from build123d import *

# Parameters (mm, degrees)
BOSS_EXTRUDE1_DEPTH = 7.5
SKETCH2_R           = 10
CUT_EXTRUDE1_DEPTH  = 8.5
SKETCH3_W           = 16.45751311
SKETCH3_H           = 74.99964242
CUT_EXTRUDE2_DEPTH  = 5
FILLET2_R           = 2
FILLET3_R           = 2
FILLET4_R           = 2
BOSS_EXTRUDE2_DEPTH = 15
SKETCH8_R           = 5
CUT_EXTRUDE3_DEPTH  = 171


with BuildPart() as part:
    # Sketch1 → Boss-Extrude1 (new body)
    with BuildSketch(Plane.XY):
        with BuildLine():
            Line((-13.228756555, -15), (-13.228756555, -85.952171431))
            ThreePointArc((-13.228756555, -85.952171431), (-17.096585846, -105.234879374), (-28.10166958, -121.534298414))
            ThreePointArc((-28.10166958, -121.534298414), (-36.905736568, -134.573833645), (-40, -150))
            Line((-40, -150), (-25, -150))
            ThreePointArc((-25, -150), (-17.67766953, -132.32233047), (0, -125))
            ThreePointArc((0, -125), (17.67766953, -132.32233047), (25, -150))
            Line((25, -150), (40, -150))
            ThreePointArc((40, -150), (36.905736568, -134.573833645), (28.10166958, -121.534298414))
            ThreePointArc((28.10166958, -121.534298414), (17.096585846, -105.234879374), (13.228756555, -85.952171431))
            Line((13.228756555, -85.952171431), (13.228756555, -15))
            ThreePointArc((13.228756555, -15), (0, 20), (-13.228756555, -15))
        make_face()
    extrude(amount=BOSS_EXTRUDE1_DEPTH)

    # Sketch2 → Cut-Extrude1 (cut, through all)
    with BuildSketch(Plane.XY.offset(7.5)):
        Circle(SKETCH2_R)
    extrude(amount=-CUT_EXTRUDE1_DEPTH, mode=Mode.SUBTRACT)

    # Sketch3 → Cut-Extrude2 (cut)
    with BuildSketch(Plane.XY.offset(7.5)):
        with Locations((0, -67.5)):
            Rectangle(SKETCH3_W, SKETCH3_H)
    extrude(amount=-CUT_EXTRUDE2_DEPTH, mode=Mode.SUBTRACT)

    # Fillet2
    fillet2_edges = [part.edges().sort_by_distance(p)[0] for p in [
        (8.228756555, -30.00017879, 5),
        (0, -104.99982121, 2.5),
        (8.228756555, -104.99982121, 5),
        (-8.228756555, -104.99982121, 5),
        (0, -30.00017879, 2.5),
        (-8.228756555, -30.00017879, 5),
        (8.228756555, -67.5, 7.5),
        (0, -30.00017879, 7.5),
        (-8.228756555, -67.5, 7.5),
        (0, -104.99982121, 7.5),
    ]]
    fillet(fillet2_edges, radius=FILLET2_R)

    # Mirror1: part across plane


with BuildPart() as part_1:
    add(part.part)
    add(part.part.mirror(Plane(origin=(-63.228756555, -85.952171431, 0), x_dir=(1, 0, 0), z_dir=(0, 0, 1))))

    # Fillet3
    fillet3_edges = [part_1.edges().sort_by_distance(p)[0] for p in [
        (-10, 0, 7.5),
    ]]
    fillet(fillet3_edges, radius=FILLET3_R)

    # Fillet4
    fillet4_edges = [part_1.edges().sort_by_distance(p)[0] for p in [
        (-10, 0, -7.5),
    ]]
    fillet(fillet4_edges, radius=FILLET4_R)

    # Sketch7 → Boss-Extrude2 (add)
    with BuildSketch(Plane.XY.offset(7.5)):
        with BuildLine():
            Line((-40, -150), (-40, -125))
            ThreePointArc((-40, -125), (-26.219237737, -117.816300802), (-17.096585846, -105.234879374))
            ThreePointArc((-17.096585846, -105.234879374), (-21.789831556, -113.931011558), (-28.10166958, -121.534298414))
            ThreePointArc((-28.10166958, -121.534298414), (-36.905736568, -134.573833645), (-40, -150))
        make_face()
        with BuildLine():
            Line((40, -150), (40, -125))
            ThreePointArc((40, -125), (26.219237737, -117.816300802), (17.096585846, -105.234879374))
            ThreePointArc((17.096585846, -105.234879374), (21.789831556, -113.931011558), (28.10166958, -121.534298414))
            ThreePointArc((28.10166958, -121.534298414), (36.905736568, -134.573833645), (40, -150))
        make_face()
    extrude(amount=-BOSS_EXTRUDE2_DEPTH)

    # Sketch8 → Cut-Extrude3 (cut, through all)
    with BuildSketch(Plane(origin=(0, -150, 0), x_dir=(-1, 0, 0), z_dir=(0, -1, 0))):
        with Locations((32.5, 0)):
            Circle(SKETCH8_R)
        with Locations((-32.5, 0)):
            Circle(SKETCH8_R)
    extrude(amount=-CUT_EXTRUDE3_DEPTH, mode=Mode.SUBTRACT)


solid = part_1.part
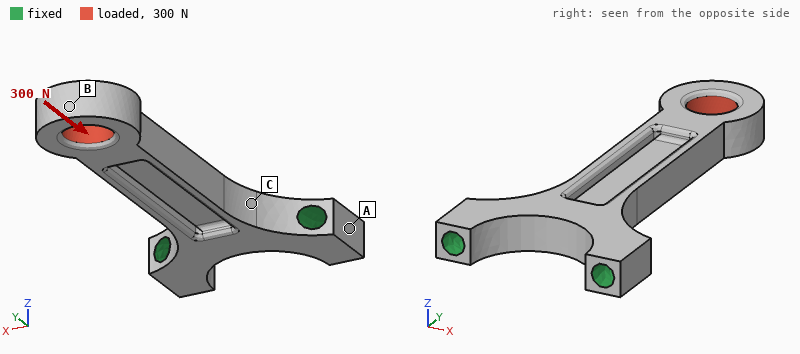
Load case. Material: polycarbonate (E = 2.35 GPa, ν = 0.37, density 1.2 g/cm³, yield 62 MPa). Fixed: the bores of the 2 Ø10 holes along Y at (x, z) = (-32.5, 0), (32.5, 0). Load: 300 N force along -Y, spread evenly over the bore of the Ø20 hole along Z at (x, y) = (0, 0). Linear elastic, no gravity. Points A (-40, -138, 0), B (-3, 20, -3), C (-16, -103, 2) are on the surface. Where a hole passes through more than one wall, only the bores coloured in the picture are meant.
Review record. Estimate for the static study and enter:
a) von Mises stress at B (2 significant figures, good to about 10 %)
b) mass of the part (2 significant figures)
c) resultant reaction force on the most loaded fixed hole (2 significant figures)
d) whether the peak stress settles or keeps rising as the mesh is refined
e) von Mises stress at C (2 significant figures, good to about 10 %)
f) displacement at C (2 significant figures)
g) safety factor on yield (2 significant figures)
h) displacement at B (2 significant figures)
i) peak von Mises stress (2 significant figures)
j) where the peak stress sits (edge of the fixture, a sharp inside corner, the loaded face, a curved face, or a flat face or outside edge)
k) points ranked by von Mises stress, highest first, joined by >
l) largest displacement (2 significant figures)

0.79 MPa
75 g
180 N
settles
1.2 MPa
13 µm
26
76 µm
2.4 MPa
the loaded face
C > B > A
78 µm
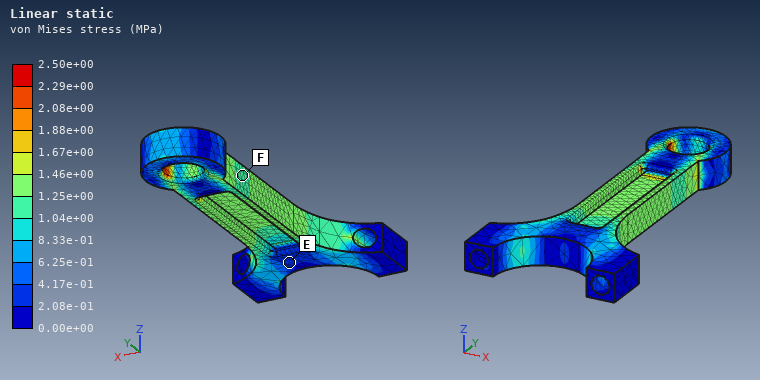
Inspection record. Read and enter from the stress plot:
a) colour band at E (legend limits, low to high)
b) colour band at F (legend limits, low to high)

2.08e-01 to 4.17e-01 MPa
1.04e+00 to 1.25e+00 MPa
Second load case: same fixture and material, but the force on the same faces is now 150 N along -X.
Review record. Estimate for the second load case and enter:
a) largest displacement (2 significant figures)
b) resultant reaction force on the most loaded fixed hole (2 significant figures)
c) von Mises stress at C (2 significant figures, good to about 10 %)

2.0 mm
410 N
7.1 MPa
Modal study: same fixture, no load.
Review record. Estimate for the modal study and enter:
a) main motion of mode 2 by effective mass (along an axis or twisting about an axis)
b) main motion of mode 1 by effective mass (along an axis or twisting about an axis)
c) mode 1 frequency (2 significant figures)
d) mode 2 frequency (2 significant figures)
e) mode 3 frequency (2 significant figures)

along X
along Z
120 Hz
330 Hz
490 Hz
